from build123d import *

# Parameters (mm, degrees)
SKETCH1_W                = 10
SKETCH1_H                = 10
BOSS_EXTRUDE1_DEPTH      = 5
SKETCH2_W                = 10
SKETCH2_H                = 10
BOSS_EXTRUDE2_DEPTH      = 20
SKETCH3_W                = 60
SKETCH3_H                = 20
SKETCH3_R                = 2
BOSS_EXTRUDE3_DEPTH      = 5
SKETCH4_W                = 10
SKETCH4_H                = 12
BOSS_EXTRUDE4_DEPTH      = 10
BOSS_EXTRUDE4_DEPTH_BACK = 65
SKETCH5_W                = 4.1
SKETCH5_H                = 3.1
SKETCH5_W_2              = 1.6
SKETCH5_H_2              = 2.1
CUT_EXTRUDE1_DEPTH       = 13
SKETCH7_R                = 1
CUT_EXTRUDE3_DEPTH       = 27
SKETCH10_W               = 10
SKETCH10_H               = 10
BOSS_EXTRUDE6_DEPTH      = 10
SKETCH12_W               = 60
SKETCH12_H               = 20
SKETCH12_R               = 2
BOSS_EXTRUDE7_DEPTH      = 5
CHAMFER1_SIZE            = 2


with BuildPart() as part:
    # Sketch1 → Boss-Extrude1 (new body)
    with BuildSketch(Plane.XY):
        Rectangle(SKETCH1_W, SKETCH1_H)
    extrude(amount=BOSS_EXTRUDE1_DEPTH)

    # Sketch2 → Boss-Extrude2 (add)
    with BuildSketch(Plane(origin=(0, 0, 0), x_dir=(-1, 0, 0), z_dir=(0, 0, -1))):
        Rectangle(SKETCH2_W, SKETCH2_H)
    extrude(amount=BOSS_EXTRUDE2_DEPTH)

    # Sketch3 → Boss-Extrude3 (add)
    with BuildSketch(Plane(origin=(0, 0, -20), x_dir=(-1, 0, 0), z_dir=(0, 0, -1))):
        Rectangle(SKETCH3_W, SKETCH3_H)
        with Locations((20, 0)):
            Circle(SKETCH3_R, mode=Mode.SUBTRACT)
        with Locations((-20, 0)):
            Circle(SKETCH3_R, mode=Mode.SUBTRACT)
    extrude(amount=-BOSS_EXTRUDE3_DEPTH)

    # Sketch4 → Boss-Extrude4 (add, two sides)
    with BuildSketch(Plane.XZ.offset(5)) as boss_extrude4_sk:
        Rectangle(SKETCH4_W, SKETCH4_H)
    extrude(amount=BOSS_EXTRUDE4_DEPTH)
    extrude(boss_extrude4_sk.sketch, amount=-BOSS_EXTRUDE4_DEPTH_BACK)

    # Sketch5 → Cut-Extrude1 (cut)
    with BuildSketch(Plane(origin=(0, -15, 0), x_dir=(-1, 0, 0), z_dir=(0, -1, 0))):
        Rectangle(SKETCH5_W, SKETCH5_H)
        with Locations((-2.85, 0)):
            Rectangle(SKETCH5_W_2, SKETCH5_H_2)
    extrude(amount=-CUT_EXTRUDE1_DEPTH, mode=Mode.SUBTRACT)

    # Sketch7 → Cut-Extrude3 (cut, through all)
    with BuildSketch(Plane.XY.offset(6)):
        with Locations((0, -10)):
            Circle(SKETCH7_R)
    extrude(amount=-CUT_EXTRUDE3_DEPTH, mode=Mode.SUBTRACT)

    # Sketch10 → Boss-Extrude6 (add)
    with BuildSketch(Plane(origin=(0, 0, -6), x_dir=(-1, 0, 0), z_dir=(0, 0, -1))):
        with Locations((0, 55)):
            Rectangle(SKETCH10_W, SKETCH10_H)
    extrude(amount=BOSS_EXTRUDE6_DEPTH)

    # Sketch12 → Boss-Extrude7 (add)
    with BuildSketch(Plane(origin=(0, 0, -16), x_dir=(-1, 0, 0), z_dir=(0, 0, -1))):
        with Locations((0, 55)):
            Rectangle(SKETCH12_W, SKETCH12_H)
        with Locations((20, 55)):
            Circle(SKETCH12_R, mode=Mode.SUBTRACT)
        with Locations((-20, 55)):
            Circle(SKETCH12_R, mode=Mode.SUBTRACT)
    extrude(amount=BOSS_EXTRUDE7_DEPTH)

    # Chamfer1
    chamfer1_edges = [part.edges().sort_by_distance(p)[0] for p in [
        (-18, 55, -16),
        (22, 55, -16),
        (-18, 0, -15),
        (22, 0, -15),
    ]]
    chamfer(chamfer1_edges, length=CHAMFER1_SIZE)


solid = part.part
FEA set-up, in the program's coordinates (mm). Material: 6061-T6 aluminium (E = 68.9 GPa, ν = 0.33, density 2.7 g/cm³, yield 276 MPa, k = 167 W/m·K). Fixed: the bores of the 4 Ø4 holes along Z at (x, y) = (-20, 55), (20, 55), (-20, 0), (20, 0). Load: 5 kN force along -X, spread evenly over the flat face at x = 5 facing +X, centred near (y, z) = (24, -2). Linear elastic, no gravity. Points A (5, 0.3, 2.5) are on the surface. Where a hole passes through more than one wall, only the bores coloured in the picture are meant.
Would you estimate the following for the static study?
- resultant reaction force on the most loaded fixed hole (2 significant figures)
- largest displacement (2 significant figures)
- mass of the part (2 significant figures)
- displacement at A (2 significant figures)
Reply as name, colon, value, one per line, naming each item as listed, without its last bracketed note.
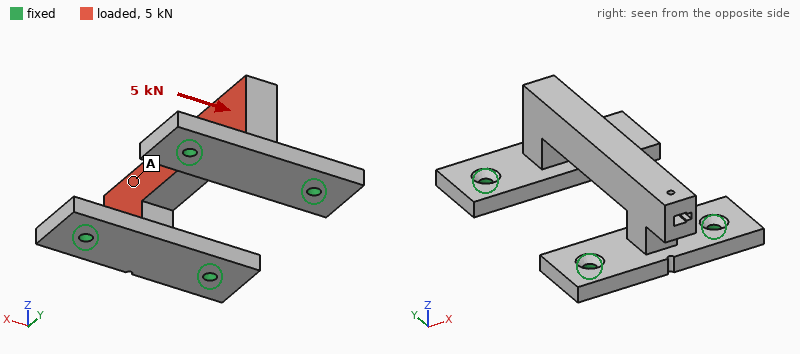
resultant reaction force on the most loaded fixed hole: 2.0 kN
largest displacement: 0.26 mm
mass of the part: 60 g
displacement at A: 0.20 mm
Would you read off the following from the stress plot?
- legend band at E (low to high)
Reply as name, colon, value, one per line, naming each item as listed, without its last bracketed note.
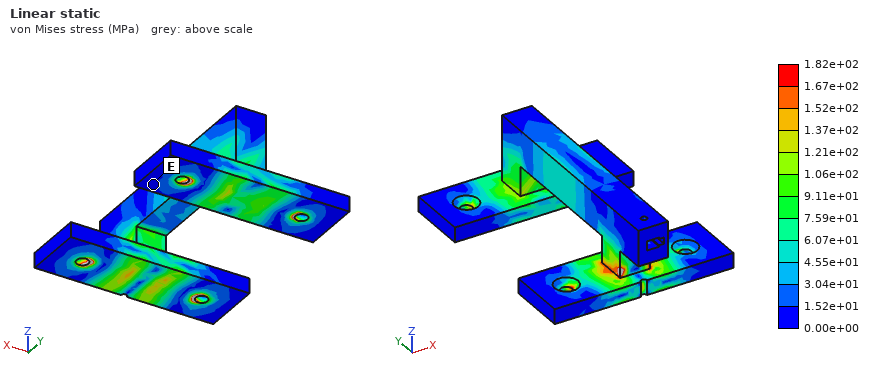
legend band at E: 0.00e+00 to 1.52e+01 MPa
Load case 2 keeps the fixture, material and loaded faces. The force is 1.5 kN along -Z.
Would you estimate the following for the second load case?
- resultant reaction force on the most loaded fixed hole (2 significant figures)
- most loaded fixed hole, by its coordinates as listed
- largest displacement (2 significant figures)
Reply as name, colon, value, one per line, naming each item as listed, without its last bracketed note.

resultant reaction force on the most loaded fixed hole: 650 N
most loaded fixed hole, by its coordinates as listed: (20, 0)
largest displacement: 47 µm
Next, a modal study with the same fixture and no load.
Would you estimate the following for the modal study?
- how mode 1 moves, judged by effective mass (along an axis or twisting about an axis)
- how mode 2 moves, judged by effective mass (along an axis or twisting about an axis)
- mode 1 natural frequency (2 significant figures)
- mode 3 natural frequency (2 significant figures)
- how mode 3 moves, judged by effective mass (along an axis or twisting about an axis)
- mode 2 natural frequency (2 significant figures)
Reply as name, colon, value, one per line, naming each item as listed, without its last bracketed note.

how mode 1 moves, judged by effective mass: along X
how mode 2 moves, judged by effective mass: along Y
mode 1 natural frequency: 4900 Hz
mode 3 natural frequency: 6500 Hz
how mode 3 moves, judged by effective mass: along Z
mode 2 natural frequency: 5600 Hz
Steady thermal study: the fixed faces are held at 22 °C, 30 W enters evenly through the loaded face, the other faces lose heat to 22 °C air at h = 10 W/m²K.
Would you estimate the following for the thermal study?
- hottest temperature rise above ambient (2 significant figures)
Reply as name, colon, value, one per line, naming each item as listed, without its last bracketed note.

hottest temperature rise above ambient: 25 K
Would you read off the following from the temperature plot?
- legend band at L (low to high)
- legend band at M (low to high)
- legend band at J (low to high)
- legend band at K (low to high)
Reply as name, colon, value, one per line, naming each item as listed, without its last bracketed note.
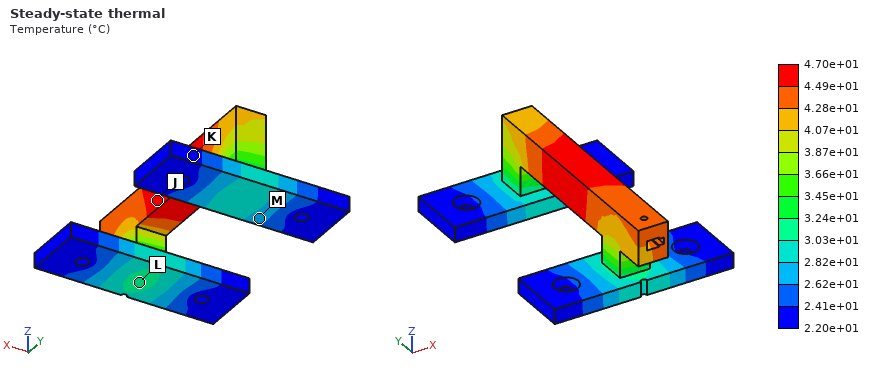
legend band at L: 3.03e+01 to 3.24e+01 °C
legend band at M: 2.62e+01 to 2.82e+01 °C
legend band at J: 4.49e+01 to 4.70e+01 °C
legend band at K: 2.20e+01 to 2.41e+01 °C
